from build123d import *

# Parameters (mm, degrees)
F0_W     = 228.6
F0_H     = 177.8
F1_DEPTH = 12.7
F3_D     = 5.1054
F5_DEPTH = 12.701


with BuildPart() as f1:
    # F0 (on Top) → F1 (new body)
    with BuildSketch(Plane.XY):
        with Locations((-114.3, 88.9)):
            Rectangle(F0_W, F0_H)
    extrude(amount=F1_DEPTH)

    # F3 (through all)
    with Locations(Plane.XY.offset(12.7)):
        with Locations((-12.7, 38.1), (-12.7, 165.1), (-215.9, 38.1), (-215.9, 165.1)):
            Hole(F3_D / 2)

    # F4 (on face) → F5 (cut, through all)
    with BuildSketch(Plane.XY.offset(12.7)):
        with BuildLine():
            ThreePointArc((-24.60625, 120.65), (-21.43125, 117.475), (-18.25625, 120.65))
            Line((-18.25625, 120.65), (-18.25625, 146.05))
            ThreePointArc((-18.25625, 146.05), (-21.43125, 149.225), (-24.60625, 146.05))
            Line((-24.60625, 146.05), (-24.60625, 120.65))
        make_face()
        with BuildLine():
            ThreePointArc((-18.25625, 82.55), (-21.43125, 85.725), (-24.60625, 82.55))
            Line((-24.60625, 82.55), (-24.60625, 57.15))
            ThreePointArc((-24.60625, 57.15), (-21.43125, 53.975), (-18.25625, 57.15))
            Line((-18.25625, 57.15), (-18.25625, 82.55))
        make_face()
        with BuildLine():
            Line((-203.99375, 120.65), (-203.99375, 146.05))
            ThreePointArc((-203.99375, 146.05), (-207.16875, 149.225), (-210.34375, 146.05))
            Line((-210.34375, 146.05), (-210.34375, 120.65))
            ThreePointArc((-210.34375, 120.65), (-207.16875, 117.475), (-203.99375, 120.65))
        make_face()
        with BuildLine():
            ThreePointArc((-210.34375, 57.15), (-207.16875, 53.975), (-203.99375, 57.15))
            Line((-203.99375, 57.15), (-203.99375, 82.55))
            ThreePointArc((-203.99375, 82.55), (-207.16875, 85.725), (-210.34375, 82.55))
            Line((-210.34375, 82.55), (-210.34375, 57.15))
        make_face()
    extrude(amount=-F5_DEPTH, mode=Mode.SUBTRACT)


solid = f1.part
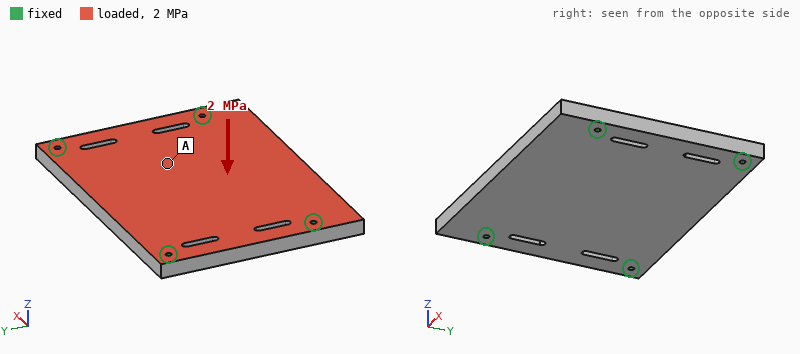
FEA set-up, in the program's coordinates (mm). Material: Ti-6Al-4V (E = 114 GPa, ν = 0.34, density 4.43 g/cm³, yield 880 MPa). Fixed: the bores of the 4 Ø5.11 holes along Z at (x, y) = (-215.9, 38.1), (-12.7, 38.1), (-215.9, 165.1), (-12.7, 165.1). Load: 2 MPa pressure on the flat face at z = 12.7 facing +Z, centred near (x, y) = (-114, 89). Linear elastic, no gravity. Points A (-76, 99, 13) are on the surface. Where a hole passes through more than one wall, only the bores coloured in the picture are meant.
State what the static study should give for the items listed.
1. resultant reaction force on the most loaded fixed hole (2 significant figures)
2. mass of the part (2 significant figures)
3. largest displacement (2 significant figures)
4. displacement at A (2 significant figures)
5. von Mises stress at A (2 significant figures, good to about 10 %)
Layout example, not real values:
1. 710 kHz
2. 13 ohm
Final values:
1. 23 kN
2. 2.2 kg
3. 0.88 mm
4. 0.72 mm
5. 110 MPa
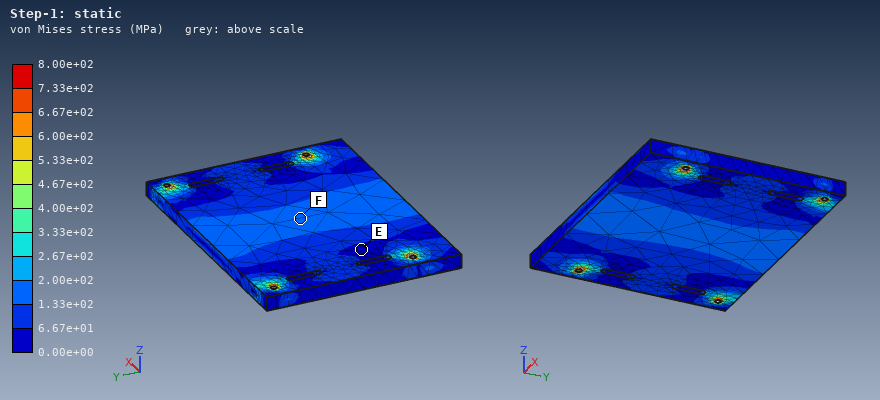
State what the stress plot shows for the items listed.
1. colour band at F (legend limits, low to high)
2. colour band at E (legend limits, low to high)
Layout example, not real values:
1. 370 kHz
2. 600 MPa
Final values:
1. 1.33e+02 to 2.00e+02 MPa
2. 0.00e+00 to 6.67e+01 MPa
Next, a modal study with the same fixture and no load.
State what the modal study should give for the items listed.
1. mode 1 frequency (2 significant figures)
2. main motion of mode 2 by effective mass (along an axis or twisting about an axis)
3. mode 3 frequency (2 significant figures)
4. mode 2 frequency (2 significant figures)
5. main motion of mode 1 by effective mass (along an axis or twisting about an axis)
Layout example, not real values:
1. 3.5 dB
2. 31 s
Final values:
1. 1200 Hz
2. twisting about X
3. 2800 Hz
4. 1600 Hz
5. along Z
